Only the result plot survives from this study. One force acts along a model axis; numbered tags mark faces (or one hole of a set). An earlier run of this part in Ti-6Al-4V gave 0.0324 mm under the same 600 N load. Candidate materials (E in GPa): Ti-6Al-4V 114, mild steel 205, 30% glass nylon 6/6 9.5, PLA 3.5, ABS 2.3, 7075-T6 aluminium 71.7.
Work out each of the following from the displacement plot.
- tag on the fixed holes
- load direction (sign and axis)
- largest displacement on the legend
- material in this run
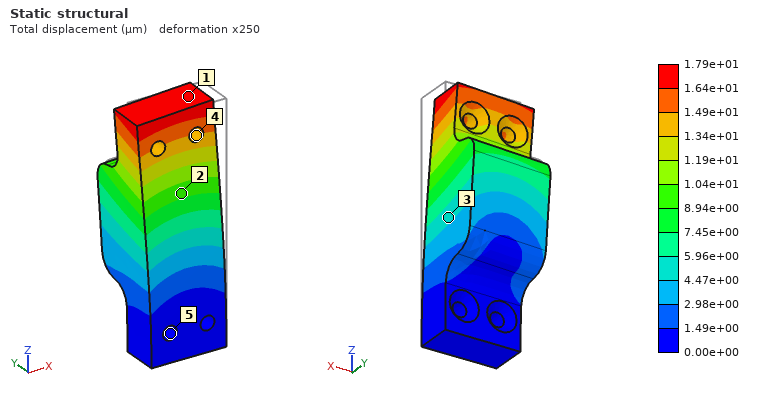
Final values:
5
-X
1.79e+01 µm
mild steel
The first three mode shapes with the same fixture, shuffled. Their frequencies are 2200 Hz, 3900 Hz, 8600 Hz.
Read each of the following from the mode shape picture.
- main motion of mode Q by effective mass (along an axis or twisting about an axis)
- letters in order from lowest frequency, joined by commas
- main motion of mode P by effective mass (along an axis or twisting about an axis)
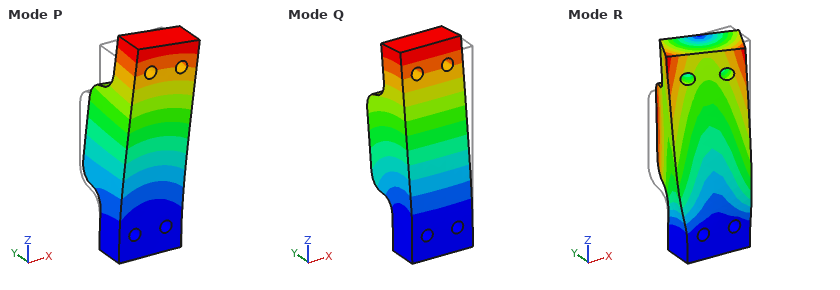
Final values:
along Y
Q, P, R
along X
